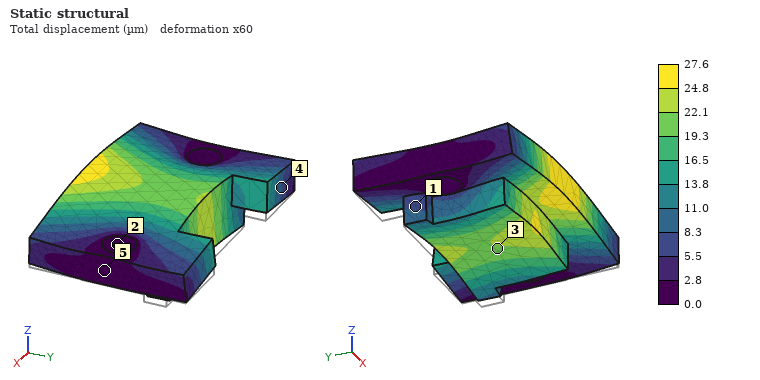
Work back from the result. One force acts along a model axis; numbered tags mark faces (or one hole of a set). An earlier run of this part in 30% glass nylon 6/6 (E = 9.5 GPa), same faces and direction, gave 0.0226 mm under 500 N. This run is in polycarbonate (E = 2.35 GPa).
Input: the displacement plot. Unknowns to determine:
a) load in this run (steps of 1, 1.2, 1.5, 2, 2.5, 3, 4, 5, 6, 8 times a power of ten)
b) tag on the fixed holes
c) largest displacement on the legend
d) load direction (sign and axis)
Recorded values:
150 N
2
27.6 µm
+Z
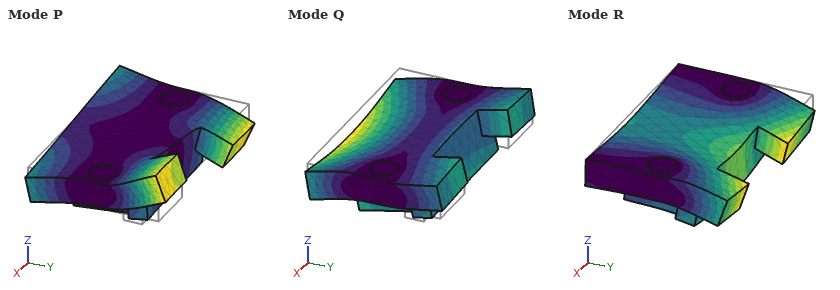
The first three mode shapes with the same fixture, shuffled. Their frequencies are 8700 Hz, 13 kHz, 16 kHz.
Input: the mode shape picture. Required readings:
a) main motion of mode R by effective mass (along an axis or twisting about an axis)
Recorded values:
along Z
